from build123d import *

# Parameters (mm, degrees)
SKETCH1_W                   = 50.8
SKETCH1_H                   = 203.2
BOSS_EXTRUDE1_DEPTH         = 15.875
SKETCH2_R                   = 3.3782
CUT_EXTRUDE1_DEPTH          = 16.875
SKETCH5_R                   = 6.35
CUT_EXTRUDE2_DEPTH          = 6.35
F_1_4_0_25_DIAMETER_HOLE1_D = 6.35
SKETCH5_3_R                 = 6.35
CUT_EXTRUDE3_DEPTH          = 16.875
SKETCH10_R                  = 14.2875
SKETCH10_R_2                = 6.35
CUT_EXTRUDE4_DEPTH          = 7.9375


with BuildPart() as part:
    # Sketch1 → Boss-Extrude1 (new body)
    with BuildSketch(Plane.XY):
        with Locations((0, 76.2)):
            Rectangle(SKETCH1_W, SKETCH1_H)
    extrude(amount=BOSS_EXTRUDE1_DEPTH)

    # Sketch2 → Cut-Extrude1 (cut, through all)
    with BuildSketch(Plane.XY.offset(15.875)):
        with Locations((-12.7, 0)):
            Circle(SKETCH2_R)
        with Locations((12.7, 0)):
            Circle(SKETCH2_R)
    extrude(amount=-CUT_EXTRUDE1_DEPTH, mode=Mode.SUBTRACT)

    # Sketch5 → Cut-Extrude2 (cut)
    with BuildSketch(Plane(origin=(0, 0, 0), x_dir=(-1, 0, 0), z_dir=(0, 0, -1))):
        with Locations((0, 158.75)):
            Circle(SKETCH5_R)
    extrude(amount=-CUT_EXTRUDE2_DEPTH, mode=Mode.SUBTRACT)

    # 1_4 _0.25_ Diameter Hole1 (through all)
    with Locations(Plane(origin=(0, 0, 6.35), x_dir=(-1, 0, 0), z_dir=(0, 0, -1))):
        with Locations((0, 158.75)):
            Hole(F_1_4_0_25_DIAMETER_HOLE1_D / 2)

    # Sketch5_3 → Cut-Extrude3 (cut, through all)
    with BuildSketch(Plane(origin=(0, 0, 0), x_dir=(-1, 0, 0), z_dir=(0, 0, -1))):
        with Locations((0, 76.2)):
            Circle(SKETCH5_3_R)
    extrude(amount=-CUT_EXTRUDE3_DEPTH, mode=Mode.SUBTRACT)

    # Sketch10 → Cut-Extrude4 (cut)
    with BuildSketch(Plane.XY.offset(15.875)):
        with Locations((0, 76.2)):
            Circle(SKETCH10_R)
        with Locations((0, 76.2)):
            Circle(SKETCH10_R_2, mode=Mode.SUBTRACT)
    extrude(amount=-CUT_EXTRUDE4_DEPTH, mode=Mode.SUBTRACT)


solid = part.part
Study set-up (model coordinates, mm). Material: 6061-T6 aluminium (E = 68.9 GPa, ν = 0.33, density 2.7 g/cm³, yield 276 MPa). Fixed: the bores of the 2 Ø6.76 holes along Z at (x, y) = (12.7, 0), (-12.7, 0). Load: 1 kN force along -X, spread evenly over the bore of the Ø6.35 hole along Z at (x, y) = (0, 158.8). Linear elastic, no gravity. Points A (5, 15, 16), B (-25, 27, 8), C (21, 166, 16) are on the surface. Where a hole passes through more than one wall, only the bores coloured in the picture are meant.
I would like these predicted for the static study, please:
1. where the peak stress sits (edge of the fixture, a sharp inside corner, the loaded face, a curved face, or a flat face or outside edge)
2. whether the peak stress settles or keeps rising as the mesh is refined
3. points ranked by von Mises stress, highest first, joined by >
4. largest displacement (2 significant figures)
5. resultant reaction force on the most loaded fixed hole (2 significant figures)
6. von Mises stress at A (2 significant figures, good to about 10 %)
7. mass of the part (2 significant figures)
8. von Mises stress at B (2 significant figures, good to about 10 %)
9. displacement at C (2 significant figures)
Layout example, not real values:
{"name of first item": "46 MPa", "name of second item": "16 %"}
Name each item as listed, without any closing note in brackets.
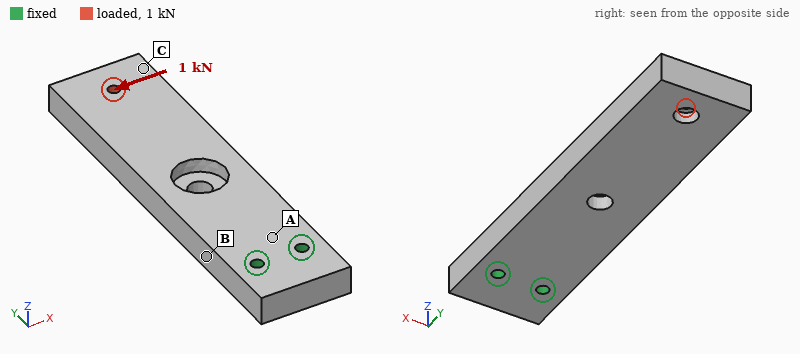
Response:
{"where the peak stress sits": "edge of the fixture", "whether the peak stress settles or keeps rising as the mesh is refined": "keeps rising", "points ranked by von Mises stress, highest first, joined by >": "B > A > C", "largest displacement": "0.17 mm", "resultant reaction force on the most loaded fixed hole": "5.5 kN", "von Mises stress at A": "8.6 MPa", "mass of the part": "420 g", "von Mises stress at B": "19 MPa", "displacement at C": "0.15 mm"}
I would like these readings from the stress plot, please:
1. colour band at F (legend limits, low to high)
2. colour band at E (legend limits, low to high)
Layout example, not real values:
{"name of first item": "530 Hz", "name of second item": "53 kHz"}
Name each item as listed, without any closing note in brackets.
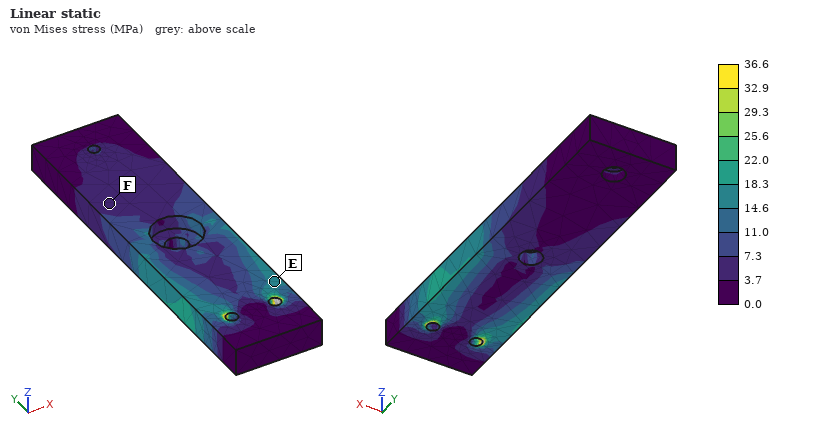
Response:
{"colour band at F": "3.7 to 7.3 MPa", "colour band at E": "14.6 to 18.3 MPa"}
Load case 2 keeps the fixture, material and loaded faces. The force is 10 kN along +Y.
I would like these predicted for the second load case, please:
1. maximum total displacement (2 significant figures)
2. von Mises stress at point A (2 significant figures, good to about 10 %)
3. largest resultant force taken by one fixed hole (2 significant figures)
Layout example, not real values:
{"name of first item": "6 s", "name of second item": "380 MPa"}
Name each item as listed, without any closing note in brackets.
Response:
{"maximum total displacement": "0.55 mm", "von Mises stress at point A": "26 MPa", "largest resultant force taken by one fixed hole": "5.0 kN"}
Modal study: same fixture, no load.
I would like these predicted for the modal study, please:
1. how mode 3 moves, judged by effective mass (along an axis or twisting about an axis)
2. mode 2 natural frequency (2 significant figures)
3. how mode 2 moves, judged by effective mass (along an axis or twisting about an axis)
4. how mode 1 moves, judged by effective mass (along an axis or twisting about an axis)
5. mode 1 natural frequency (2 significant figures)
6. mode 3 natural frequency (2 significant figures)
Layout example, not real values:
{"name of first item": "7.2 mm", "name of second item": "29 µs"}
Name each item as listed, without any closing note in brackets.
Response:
{"how mode 3 moves, judged by effective mass": "twisting about Y", "mode 2 natural frequency": "1200 Hz", "how mode 2 moves, judged by effective mass": "along X", "how mode 1 moves, judged by effective mass": "along Z", "mode 1 natural frequency": "400 Hz", "mode 3 natural frequency": "2300 Hz"}
